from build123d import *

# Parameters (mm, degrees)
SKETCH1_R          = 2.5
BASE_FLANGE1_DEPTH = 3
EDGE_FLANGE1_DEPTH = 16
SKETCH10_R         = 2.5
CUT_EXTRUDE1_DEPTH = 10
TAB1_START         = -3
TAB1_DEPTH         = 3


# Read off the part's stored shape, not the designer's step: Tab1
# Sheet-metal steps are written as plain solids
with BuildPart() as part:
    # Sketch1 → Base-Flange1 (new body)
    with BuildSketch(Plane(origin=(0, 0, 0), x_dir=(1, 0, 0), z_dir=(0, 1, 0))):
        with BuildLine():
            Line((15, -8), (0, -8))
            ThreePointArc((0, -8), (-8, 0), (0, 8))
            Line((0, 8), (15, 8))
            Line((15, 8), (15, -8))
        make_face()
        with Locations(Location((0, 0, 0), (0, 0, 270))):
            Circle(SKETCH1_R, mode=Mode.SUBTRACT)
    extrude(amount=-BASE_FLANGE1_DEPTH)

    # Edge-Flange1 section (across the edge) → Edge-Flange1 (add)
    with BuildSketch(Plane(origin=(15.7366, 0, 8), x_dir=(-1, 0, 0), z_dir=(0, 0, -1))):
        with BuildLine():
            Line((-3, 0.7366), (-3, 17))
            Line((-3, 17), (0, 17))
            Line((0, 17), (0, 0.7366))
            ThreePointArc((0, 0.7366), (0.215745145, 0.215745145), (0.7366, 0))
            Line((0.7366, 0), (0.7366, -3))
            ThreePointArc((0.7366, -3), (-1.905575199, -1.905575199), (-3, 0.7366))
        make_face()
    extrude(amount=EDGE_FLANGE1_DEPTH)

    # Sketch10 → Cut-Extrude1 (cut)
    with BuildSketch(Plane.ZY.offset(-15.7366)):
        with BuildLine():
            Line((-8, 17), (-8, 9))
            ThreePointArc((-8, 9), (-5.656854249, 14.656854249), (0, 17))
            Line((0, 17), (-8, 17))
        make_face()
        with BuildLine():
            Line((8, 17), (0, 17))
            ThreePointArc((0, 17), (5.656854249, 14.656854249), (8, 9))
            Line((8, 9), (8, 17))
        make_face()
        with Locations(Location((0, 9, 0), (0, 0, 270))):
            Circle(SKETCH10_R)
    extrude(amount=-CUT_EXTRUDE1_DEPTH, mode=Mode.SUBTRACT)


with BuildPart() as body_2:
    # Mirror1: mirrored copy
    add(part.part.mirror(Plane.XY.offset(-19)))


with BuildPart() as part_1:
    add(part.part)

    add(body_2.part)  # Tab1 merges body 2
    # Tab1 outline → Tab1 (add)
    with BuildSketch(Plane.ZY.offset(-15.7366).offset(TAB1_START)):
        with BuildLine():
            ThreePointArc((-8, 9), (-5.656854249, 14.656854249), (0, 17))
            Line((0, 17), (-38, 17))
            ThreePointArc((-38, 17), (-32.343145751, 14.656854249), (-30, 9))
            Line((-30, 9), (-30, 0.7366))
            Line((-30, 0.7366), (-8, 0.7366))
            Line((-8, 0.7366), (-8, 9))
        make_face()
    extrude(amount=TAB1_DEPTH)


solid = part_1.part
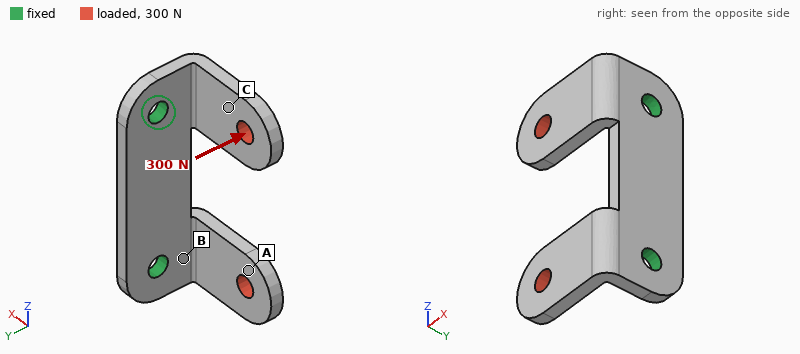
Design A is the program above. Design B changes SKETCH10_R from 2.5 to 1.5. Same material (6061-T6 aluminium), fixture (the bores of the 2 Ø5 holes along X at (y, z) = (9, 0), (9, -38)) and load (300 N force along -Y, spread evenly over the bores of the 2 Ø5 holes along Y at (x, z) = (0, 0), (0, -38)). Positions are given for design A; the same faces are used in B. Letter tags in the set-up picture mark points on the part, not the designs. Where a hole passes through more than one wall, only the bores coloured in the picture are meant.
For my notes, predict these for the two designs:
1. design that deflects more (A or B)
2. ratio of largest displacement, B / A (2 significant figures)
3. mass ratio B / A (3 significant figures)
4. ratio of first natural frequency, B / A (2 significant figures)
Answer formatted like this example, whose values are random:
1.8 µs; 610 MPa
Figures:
B; 1.1; 1.02; 0.94
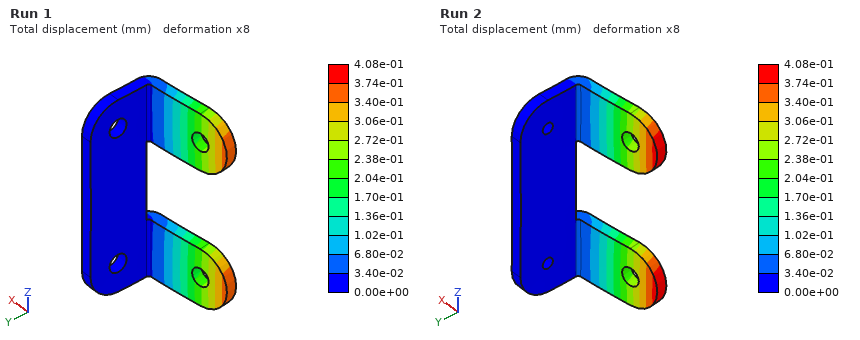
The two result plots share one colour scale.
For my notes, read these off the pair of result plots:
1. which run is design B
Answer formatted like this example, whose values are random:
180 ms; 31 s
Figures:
Run 2
